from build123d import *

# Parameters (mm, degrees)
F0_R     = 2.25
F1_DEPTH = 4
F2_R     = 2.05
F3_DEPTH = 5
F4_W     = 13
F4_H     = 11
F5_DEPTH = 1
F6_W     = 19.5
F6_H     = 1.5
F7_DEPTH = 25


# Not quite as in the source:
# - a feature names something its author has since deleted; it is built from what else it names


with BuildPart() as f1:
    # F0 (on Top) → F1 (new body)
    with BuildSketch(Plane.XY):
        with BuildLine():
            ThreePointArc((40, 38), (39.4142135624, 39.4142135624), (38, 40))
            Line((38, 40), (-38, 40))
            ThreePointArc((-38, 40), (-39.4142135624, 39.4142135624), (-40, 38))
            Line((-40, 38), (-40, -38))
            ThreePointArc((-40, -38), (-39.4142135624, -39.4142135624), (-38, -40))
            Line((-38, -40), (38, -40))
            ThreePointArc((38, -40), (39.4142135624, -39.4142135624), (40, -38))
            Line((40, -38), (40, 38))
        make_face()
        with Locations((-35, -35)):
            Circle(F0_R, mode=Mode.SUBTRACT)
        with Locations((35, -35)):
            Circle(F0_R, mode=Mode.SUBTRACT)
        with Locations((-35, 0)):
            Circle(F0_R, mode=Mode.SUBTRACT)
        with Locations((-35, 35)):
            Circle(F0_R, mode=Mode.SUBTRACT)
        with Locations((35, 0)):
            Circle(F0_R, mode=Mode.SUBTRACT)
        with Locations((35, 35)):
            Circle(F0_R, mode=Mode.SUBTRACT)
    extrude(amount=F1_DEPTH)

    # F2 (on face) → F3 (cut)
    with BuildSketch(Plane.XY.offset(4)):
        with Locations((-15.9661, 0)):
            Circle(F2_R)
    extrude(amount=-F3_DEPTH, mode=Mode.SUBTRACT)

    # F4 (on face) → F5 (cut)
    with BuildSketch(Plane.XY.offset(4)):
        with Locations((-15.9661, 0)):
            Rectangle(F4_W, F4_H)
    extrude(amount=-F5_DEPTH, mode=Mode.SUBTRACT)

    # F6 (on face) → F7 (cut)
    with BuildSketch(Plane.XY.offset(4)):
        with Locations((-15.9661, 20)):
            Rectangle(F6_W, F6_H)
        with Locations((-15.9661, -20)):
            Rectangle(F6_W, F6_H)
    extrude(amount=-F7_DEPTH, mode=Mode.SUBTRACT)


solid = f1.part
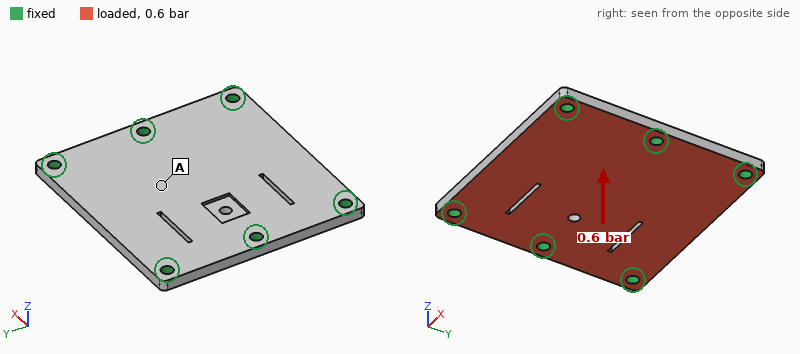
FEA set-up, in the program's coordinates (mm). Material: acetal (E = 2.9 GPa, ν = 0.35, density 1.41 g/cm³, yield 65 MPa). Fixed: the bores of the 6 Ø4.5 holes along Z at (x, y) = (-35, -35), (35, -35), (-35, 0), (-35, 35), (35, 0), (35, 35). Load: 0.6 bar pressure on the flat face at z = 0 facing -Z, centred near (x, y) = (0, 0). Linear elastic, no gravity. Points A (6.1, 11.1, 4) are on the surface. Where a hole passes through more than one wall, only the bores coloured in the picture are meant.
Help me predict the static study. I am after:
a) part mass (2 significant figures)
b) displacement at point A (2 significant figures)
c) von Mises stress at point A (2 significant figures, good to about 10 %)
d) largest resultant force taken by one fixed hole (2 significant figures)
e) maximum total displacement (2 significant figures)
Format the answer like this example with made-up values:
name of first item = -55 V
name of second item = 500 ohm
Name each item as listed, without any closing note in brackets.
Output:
part mass = 35 g
displacement at point A = 0.27 mm
von Mises stress at point A = 3.9 MPa
largest resultant force taken by one fixed hole = 85 N
maximum total displacement = 0.29 mm
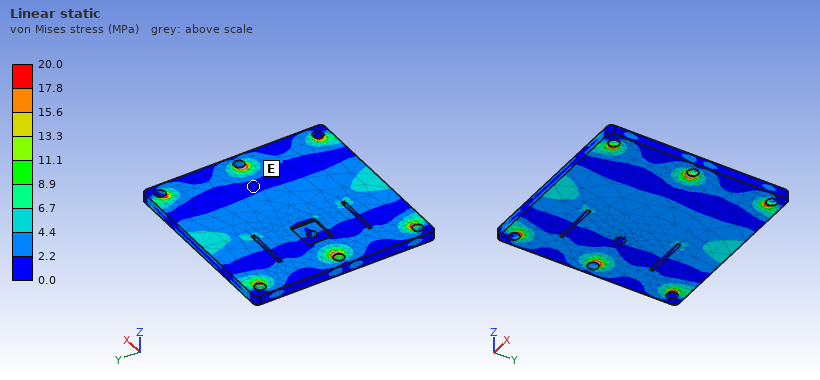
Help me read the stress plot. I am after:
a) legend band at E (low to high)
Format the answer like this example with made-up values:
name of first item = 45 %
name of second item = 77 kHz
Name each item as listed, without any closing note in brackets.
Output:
legend band at E = 0.0 to 2.2 MPa
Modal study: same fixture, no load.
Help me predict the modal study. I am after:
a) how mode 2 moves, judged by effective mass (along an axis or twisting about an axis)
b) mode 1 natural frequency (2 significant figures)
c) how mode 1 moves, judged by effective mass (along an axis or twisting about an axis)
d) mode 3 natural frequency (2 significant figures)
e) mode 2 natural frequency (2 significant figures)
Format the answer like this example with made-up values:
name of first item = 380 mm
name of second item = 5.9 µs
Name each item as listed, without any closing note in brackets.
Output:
how mode 2 moves, judged by effective mass = twisting about X
mode 1 natural frequency = 1100 Hz
how mode 1 moves, judged by effective mass = along Z
mode 3 natural frequency = 2000 Hz
mode 2 natural frequency = 1300 Hz
